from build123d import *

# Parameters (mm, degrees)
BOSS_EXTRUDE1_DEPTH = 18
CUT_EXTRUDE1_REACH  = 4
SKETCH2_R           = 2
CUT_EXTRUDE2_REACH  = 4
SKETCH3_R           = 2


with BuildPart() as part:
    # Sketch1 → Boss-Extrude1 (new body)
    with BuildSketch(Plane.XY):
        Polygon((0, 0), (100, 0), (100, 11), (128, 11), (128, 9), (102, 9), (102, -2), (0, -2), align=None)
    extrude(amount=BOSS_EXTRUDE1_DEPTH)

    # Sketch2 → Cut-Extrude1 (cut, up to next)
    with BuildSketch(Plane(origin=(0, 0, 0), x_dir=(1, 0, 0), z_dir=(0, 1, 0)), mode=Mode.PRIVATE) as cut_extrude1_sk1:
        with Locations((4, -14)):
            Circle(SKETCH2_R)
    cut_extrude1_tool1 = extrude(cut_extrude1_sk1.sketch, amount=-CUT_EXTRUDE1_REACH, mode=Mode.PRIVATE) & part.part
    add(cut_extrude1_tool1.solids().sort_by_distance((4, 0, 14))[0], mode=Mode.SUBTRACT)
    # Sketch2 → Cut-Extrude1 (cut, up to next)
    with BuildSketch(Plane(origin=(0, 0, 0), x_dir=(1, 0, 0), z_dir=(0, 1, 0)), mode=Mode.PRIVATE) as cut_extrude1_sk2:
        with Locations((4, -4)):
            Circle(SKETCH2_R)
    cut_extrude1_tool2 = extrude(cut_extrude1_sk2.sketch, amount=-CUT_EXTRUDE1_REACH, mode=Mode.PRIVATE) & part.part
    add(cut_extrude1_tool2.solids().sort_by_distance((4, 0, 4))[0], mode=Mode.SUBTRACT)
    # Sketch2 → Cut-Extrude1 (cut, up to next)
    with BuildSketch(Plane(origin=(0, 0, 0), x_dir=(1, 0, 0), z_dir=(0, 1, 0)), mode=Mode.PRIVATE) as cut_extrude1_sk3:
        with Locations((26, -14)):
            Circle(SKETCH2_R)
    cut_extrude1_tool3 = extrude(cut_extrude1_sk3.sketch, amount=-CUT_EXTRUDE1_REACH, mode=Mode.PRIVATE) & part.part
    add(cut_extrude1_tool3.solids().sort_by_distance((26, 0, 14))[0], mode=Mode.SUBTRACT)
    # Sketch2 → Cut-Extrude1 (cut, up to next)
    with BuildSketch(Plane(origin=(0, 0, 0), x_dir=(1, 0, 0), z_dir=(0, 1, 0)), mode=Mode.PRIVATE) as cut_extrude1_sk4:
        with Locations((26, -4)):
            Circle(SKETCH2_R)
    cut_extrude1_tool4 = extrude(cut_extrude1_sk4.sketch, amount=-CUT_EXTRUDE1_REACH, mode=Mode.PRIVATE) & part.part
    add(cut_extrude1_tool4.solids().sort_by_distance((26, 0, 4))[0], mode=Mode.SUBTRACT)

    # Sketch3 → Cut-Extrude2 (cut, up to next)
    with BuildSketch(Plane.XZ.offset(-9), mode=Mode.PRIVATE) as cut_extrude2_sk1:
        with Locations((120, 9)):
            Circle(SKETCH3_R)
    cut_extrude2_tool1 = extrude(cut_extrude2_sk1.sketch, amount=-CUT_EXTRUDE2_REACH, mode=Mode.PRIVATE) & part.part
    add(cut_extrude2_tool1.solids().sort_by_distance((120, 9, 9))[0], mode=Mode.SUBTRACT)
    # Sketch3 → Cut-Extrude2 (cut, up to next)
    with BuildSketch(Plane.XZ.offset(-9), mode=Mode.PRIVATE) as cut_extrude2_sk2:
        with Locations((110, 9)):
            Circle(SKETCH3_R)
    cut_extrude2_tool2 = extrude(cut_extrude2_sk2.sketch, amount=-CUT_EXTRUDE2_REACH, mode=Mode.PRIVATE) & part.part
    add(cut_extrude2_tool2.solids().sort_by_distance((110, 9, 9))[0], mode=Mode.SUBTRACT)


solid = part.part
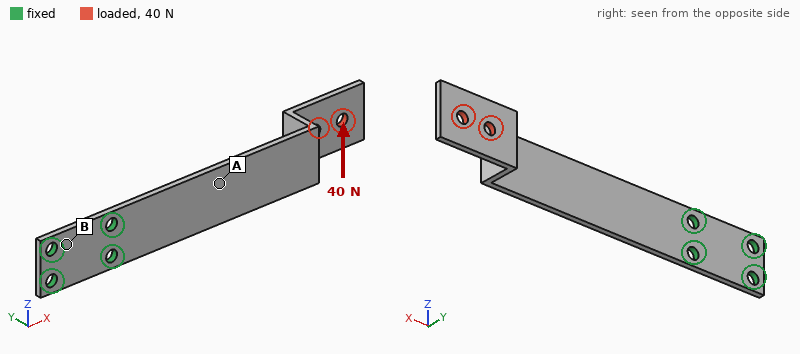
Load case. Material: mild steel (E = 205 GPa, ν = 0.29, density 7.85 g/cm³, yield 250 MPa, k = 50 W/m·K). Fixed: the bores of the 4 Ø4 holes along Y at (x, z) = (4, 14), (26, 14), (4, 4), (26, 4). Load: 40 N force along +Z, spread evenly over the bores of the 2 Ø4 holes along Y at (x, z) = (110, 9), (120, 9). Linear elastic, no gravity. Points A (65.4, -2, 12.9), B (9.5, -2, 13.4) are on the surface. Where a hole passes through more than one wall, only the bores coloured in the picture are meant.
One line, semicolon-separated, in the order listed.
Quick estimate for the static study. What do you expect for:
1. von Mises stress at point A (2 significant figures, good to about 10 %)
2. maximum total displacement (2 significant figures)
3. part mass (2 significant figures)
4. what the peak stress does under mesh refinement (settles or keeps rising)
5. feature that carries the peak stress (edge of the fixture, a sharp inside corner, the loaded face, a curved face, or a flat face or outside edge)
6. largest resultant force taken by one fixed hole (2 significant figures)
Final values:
33 MPa; 0.19 mm; 38 g; keeps rising; edge of the fixture; 290 N
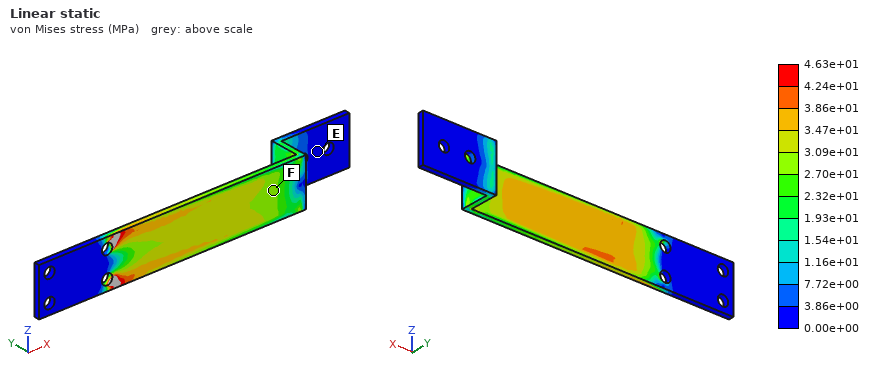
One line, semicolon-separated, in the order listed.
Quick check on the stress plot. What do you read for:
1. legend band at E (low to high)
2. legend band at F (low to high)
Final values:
0.00e+00 to 3.86e+00 MPa; 2.70e+01 to 3.09e+01 MPa
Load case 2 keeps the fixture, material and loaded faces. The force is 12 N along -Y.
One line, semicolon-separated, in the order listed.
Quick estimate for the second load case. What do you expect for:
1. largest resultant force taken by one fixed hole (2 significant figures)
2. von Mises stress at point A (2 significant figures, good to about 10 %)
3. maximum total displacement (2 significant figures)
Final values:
6.1 N; 50 MPa; 1.4 mm
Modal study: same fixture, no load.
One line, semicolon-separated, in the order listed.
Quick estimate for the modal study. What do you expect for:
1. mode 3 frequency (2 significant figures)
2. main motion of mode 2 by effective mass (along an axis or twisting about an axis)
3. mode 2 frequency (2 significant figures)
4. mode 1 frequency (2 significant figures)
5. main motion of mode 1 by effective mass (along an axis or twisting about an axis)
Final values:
900 Hz; along Z; 830 Hz; 150 Hz; along Y
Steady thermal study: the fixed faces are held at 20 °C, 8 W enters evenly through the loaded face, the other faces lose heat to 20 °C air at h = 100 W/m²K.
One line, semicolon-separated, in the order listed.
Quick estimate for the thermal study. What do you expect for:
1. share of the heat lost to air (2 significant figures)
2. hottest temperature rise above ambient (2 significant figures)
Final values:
99 %; 60 K
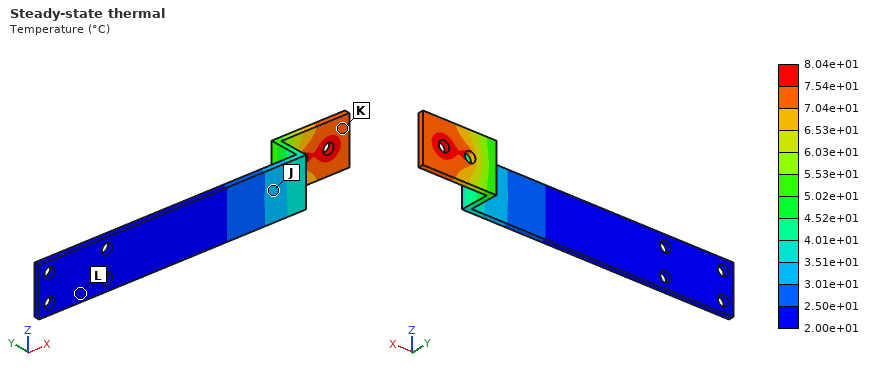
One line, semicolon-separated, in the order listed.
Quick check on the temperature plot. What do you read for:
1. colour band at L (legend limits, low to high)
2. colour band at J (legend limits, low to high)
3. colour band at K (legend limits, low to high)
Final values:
2.00e+01 to 2.50e+01 °C; 3.01e+01 to 3.51e+01 °C; 7.04e+01 to 7.54e+01 °C
